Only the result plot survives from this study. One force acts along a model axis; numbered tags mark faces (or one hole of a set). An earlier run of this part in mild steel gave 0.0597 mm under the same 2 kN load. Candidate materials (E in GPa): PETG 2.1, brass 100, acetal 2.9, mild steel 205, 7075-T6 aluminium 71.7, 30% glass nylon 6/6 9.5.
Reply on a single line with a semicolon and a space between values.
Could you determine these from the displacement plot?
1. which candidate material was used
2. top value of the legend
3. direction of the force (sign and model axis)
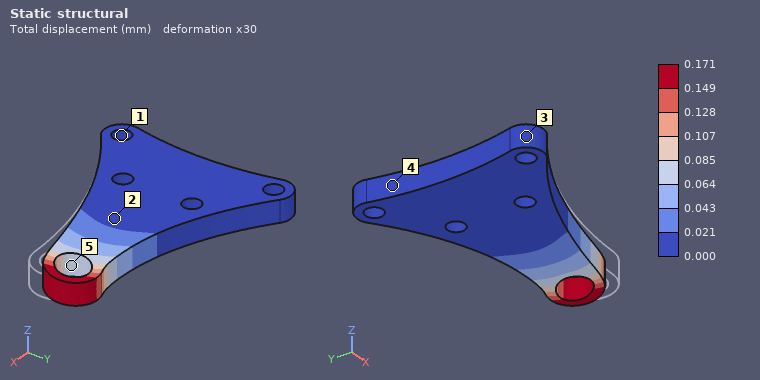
7075-T6 aluminium; 0.171 mm; +Y
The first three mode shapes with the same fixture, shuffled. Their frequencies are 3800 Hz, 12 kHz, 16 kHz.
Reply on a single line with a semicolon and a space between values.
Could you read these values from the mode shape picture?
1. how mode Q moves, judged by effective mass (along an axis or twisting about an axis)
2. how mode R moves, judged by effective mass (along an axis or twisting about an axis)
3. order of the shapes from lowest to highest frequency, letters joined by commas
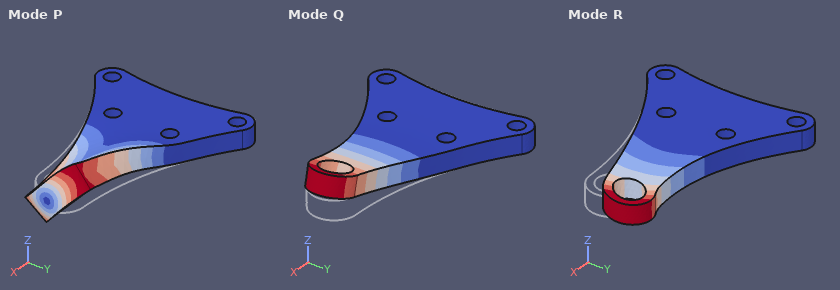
along Z; along Y; Q, R, P
